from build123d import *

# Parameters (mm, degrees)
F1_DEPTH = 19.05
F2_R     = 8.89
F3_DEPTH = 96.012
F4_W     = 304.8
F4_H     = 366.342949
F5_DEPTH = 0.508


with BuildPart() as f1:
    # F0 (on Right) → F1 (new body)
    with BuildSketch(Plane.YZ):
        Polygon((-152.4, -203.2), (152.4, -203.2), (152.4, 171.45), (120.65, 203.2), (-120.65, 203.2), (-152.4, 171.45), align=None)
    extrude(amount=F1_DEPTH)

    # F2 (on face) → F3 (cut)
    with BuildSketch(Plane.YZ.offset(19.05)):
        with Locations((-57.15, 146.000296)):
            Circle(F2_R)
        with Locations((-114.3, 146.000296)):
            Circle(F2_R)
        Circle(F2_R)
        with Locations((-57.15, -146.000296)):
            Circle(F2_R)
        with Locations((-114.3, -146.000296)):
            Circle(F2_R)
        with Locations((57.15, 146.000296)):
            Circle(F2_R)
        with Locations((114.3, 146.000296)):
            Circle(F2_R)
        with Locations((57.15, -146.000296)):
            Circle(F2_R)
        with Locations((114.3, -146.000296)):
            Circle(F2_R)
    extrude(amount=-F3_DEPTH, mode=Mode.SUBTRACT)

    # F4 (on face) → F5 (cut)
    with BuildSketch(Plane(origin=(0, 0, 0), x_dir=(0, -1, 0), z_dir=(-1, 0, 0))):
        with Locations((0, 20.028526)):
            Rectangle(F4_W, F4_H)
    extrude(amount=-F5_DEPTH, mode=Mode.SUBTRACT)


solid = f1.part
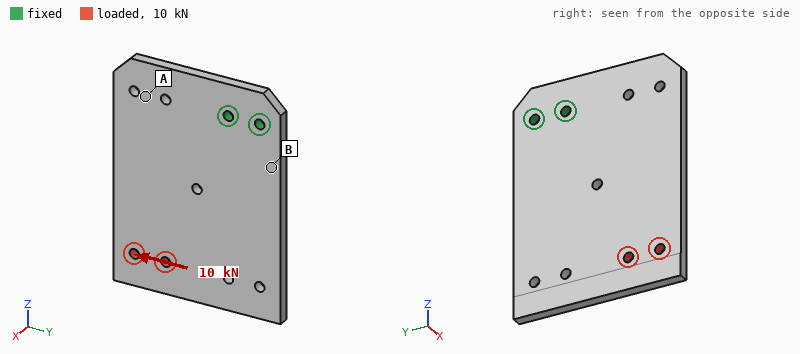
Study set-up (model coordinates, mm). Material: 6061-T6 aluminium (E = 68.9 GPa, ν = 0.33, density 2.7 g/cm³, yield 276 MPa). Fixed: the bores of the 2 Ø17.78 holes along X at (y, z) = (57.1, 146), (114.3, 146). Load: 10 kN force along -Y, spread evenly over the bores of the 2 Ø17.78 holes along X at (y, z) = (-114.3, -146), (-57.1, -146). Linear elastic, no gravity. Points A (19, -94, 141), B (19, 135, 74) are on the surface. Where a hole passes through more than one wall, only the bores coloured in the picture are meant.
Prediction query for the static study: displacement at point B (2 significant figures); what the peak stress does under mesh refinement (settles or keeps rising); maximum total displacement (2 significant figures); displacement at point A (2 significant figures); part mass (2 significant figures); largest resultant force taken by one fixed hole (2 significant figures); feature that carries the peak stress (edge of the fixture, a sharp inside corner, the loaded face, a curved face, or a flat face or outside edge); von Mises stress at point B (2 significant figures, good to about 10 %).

0.075 mm
keeps rising
0.43 mm
0.16 mm
6.1 kg
41 kN
edge of the fixture
17 MPa
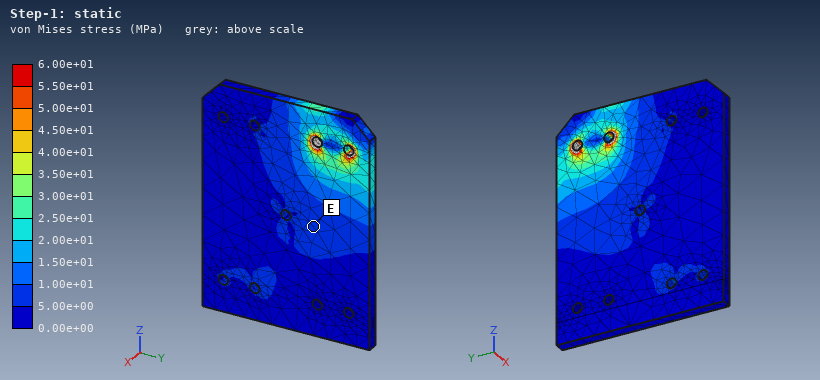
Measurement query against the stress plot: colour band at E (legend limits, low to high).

5.00e+00 to 1.00e+01 MPa
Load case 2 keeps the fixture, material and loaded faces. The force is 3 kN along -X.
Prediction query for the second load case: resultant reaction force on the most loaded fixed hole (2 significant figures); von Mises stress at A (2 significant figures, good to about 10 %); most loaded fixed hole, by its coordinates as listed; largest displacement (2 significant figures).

6.6 kN
28 MPa
(57.1, 146)
5.5 mm
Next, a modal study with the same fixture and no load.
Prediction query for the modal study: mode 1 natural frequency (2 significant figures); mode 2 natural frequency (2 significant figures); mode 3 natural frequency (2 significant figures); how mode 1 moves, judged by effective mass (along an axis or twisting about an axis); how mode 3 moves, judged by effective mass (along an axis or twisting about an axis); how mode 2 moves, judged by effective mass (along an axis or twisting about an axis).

100 Hz
230 Hz
480 Hz
along X
along X
twisting about Z
